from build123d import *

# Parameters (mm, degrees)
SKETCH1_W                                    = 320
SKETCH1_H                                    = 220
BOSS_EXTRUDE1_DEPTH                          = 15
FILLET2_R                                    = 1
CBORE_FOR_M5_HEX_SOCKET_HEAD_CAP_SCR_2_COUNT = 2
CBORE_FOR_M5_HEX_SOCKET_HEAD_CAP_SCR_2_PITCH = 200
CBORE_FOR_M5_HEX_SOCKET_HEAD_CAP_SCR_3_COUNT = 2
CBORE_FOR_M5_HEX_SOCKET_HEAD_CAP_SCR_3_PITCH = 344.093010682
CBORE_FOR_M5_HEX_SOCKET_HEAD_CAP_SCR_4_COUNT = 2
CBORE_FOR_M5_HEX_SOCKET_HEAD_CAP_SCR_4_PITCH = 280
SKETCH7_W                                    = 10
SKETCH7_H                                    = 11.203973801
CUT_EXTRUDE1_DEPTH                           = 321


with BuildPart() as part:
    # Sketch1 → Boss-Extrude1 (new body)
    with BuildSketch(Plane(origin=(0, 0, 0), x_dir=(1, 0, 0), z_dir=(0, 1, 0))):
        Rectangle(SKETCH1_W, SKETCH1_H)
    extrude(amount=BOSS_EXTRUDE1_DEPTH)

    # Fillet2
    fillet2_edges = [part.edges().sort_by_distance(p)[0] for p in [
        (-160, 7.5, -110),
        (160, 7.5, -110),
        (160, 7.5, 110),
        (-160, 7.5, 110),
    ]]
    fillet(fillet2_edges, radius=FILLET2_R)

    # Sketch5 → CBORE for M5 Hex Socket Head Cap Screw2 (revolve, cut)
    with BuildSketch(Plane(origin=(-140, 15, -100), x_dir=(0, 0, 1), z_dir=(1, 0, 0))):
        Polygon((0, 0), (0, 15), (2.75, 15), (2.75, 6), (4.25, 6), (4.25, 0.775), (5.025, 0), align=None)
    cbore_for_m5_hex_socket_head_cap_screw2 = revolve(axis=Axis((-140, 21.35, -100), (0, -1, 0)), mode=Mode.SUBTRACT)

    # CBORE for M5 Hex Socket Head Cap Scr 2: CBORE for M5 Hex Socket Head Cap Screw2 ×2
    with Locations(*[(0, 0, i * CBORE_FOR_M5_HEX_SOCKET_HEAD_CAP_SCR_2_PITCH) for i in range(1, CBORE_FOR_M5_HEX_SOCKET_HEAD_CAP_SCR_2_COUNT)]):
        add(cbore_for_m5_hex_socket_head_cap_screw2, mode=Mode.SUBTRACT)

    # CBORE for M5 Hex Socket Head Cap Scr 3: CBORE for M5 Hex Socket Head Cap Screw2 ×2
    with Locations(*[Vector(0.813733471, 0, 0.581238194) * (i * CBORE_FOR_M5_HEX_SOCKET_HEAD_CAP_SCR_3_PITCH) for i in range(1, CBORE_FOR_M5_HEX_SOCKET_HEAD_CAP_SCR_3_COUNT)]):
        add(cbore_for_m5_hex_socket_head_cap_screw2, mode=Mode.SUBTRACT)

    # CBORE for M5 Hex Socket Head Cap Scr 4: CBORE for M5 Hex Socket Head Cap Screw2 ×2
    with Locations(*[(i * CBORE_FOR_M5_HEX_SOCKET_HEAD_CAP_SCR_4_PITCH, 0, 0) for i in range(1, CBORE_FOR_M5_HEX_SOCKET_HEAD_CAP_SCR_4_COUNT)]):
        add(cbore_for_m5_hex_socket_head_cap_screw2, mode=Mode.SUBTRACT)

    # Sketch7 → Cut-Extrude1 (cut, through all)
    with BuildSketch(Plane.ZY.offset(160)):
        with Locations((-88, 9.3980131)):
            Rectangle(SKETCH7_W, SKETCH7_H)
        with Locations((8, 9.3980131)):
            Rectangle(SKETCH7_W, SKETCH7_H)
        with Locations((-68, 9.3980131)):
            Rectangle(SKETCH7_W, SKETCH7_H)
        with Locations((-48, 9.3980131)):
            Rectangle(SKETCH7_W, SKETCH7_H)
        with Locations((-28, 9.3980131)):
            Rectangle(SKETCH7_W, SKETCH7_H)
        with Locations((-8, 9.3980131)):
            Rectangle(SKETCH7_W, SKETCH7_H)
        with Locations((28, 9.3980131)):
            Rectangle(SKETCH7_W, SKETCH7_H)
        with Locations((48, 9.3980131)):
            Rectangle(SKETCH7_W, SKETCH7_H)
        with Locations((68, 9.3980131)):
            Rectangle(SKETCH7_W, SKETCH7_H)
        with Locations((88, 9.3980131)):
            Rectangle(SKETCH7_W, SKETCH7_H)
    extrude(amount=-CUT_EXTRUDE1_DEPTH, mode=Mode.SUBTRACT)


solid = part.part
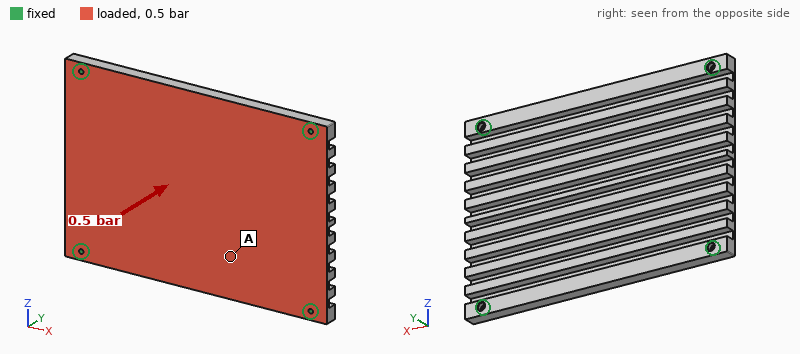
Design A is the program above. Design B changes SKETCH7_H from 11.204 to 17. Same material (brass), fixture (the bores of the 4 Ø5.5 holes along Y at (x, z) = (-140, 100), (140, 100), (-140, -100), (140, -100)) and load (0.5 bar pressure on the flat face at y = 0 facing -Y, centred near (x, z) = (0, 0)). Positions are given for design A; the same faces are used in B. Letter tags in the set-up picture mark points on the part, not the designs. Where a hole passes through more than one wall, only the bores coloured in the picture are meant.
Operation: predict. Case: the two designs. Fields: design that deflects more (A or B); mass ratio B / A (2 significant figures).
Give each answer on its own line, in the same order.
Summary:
B
0.87
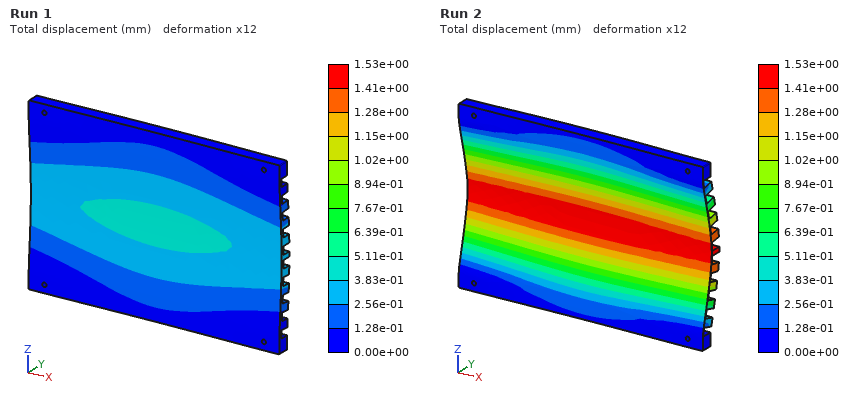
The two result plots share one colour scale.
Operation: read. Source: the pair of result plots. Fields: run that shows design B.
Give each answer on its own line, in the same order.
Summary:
Run 2
